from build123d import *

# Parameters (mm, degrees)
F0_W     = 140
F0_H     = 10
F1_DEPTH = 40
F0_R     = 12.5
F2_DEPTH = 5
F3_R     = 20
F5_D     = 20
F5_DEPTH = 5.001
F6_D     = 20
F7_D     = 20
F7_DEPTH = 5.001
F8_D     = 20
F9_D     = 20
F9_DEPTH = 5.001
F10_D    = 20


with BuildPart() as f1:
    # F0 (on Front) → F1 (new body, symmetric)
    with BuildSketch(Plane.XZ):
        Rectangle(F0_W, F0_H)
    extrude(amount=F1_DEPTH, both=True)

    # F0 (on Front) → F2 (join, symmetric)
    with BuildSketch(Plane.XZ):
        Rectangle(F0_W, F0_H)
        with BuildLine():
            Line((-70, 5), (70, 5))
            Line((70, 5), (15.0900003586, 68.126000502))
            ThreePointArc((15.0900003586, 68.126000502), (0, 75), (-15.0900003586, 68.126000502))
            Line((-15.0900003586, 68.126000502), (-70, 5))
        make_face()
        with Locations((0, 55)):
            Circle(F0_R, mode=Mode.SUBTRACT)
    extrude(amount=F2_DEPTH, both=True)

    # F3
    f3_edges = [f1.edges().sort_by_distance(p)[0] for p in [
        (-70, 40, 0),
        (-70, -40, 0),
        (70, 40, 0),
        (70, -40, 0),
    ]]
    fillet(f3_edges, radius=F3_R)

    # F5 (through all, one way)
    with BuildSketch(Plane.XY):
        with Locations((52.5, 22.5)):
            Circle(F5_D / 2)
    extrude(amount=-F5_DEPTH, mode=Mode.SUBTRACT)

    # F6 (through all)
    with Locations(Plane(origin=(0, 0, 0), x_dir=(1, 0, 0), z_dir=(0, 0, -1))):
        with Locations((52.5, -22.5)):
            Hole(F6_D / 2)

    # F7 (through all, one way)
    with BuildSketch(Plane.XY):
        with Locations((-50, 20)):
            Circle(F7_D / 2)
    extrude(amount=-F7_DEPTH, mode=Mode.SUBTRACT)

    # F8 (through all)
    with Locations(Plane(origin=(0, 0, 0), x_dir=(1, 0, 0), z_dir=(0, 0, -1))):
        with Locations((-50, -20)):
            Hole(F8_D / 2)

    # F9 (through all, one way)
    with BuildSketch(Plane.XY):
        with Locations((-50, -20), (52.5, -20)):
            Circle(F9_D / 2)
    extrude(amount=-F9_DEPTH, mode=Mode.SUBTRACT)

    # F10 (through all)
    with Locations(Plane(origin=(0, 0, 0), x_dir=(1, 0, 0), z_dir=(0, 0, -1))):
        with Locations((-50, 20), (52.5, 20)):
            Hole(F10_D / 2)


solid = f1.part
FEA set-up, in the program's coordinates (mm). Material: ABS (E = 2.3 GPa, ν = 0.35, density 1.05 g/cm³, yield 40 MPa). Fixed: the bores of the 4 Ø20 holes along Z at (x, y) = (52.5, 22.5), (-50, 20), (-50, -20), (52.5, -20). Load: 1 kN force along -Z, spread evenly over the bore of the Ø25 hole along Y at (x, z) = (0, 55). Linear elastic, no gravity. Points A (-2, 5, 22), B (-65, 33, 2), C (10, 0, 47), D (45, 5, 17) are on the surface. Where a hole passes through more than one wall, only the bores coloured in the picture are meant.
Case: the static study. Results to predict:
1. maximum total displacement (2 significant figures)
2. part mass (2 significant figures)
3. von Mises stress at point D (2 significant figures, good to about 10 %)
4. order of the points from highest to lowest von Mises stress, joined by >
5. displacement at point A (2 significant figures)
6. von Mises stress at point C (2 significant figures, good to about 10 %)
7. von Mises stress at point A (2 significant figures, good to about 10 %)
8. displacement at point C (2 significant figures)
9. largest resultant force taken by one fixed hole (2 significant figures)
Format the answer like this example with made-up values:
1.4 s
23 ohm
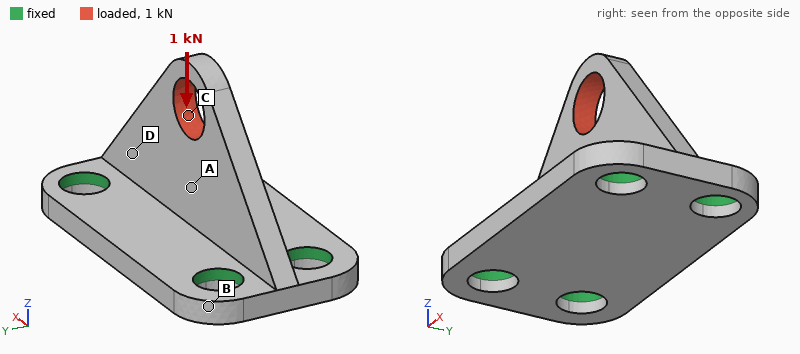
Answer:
0.11 mm
150 g
1.6 MPa
C > D > A > B
0.065 mm
2.2 MPa
0.80 MPa
0.075 mm
280 N
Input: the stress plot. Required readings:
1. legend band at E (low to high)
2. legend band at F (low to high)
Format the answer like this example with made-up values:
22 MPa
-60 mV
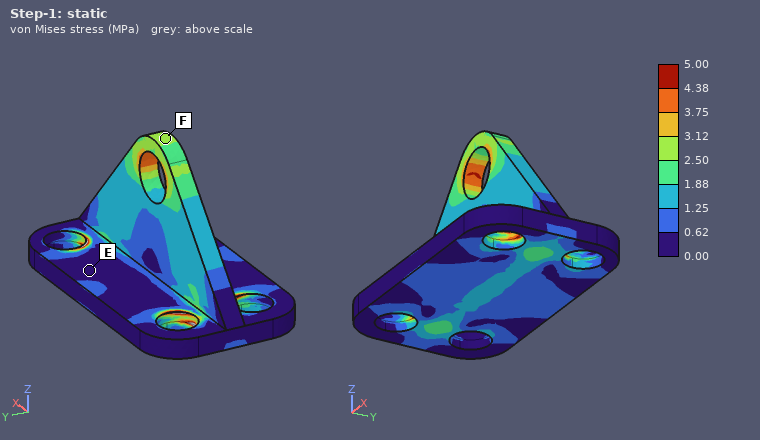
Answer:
0.00 to 0.62 MPa
2.50 to 3.12 MPa
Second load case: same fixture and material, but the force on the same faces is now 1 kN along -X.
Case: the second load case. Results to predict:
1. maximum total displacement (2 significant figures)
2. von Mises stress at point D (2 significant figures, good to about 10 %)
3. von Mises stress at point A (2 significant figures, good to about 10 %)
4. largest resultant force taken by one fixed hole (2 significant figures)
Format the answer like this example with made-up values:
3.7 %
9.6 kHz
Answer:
0.22 mm
2.3 MPa
1.8 MPa
390 N
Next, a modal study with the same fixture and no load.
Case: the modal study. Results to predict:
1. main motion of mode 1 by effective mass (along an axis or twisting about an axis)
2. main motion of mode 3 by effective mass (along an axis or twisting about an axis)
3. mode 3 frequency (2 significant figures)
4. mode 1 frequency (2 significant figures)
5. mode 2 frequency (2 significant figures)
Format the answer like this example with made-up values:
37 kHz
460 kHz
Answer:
along Y
along Z
2000 Hz
720 Hz
1700 Hz
